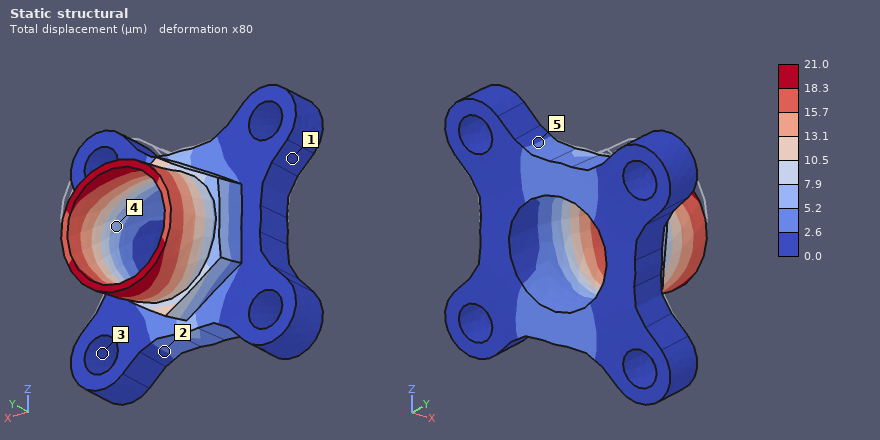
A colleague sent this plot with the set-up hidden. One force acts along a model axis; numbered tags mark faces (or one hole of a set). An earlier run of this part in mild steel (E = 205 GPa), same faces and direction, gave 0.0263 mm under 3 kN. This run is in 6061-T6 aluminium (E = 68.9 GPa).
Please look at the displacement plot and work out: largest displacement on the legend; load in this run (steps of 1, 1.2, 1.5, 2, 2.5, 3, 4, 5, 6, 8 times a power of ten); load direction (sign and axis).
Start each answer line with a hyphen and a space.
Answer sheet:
- 21.0 µm
- 800 N
- -Z
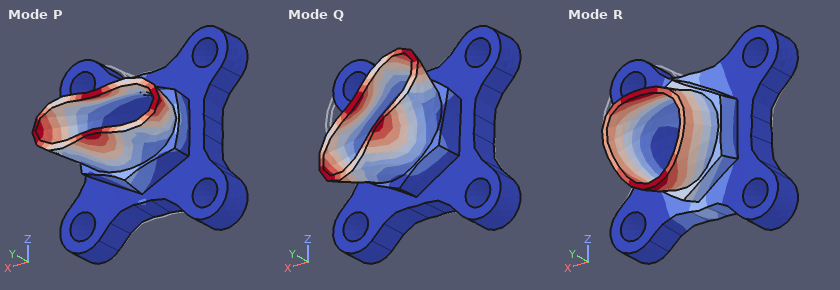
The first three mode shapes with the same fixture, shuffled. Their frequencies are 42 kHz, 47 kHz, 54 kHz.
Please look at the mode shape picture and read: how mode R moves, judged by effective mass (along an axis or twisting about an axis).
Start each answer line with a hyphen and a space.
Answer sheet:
- along Z
